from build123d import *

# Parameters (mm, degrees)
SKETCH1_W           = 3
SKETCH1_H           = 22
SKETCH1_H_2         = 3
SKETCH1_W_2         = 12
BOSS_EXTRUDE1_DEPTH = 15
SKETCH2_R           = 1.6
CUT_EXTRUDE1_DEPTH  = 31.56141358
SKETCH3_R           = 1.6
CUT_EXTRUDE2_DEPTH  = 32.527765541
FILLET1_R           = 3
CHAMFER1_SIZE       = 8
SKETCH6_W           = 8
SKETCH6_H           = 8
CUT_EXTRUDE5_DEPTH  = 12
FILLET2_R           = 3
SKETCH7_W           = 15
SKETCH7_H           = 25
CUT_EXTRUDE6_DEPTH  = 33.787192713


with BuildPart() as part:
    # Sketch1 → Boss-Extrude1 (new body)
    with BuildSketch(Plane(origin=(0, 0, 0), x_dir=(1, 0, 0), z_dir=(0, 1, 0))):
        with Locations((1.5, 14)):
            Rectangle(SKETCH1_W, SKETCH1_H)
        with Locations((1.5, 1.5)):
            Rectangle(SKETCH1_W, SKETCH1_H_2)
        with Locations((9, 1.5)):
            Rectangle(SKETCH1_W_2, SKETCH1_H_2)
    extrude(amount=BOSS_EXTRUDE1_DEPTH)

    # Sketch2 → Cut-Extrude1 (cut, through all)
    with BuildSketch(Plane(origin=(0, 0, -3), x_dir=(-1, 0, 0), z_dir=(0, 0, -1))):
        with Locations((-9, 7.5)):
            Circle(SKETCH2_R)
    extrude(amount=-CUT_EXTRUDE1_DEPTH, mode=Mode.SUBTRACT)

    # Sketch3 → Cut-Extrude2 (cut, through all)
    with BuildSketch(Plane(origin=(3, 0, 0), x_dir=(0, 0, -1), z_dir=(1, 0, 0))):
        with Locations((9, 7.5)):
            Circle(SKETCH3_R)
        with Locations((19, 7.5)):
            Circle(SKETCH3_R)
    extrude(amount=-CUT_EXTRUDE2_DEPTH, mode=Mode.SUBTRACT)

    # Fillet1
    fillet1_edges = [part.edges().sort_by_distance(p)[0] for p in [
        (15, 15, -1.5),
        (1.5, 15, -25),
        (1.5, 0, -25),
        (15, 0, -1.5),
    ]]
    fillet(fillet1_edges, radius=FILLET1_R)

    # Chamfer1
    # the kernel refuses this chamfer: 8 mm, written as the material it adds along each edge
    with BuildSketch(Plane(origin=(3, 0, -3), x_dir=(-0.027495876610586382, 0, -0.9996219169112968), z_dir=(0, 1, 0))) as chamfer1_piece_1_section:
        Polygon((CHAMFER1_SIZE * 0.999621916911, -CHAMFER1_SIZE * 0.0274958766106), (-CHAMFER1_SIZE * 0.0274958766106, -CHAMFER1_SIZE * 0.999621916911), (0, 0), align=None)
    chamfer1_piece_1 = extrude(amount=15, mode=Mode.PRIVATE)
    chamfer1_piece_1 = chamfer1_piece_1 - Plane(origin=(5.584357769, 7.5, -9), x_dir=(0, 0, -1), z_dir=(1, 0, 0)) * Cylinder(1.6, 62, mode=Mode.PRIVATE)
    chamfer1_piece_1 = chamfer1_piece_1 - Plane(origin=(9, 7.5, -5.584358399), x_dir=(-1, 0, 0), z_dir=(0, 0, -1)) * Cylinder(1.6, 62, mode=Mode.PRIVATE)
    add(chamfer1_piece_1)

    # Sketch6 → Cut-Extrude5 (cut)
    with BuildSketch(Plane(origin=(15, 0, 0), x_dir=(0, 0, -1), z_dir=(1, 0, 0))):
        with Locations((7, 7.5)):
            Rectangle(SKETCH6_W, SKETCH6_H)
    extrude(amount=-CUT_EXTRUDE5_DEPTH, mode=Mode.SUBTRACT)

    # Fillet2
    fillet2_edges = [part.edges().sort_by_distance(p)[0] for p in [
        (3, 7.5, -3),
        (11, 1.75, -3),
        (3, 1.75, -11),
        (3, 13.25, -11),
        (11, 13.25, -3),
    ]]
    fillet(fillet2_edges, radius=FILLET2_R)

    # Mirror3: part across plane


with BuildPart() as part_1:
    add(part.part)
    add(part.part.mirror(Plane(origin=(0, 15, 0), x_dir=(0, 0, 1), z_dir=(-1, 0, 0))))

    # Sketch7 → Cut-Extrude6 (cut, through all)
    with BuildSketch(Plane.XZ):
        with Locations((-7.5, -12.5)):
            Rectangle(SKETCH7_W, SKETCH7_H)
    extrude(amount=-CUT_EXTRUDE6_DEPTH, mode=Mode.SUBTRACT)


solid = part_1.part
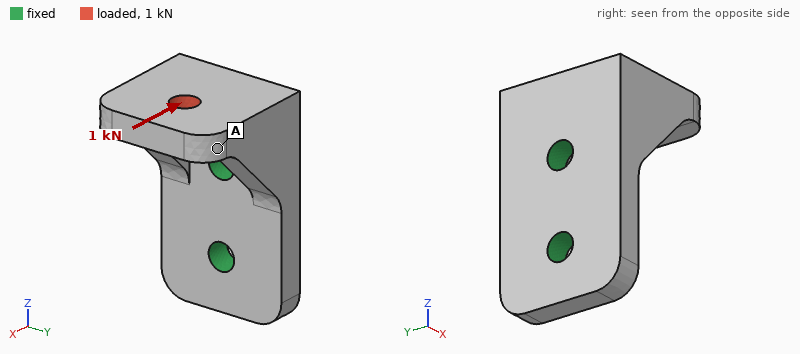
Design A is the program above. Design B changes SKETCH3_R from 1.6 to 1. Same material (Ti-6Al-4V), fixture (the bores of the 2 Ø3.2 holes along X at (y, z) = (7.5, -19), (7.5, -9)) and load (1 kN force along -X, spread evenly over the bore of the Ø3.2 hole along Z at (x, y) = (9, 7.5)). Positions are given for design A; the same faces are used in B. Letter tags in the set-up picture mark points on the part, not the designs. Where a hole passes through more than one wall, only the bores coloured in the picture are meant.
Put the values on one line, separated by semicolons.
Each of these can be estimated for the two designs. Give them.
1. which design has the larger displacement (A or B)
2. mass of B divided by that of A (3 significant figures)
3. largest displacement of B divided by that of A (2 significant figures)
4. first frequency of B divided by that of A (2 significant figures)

B; 1.02; 1.3; 0.87
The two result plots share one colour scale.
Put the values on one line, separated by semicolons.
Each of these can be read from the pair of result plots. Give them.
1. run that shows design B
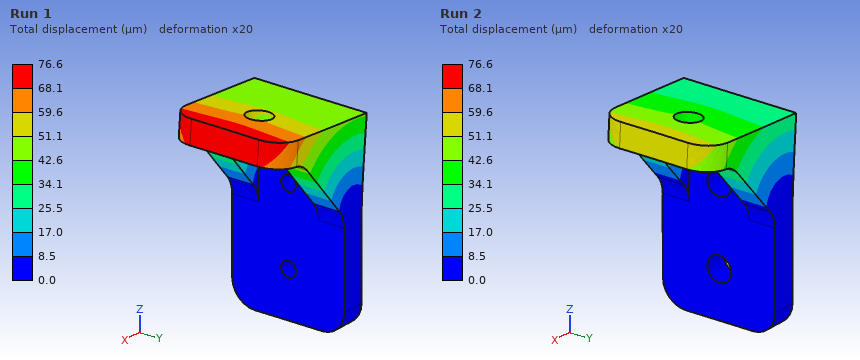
Run 1
